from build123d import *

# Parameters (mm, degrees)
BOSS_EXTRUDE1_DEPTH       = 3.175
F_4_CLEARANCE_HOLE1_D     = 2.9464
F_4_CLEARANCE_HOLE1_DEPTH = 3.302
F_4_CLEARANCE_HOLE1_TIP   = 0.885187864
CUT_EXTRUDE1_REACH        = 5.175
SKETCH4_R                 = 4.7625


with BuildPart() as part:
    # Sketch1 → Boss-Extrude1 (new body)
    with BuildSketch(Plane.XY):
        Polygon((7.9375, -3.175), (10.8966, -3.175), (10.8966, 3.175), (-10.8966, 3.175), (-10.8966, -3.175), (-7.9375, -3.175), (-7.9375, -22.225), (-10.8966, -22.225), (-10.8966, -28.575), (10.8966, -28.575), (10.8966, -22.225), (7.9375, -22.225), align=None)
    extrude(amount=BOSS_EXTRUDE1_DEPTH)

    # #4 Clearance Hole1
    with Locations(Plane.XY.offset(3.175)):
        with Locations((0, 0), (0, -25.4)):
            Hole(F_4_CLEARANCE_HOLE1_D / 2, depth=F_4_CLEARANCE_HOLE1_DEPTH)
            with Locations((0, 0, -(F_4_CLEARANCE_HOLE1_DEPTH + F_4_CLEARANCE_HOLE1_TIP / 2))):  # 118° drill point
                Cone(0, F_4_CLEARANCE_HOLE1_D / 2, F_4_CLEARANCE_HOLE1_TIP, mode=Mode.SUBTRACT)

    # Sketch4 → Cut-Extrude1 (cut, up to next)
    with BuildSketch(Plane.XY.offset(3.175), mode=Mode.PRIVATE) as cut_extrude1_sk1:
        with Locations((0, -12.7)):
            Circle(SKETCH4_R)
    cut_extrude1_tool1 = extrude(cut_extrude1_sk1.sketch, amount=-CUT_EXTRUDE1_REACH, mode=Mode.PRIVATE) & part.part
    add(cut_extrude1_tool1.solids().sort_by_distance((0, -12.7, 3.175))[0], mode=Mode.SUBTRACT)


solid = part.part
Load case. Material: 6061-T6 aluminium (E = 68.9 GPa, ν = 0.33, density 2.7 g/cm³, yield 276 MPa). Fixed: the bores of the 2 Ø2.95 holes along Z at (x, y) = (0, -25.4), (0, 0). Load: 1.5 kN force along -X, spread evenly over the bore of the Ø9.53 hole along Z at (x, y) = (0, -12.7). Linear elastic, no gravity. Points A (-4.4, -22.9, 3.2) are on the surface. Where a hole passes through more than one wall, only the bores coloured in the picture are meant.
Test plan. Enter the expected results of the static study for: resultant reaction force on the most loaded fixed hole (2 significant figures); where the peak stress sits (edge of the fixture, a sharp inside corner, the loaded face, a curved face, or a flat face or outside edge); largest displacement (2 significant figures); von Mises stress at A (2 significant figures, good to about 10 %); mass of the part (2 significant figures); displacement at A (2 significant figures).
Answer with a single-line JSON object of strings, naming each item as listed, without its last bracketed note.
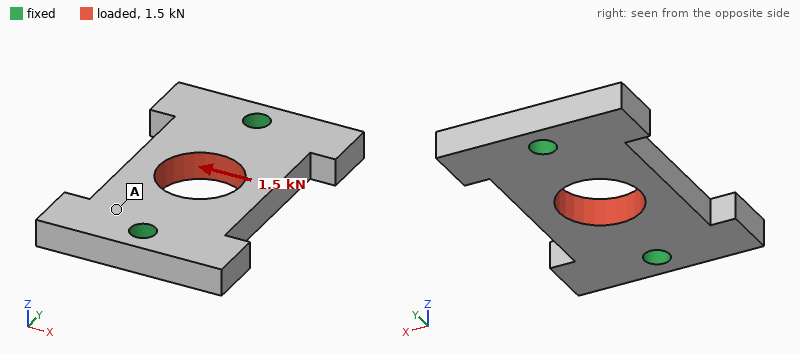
{"resultant reaction force on the most loaded fixed hole": "750 N", "where the peak stress sits": "edge of the fixture", "largest displacement": "13 µm", "von Mises stress at A": "21 MPa", "mass of the part": "4.2 g", "displacement at A": "3.7 µm"}
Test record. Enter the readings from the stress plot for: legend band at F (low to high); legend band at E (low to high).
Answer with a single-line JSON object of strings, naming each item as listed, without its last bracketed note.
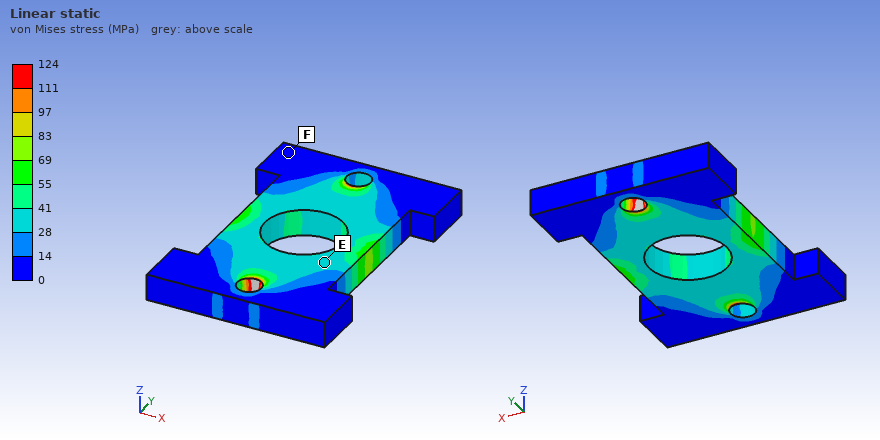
{"legend band at F": "0 to 14 MPa", "legend band at E": "28 to 41 MPa"}
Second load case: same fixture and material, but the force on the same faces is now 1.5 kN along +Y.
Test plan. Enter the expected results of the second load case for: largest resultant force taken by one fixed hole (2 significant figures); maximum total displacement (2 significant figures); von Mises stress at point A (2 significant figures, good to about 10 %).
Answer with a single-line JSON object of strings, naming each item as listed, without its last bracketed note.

{"largest resultant force taken by one fixed hole": "750 N", "maximum total displacement": "4.5 µm", "von Mises stress at point A": "13 MPa"}
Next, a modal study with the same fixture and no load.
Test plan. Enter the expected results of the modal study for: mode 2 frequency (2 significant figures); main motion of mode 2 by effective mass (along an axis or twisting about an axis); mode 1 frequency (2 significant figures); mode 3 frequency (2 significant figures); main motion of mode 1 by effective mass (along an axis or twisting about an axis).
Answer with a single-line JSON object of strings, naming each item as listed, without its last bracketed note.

{"mode 2 frequency": "22 kHz", "main motion of mode 2 by effective mass": "along Z", "mode 1 frequency": "19 kHz", "mode 3 frequency": "26 kHz", "main motion of mode 1 by effective mass": "twisting about Y"}
